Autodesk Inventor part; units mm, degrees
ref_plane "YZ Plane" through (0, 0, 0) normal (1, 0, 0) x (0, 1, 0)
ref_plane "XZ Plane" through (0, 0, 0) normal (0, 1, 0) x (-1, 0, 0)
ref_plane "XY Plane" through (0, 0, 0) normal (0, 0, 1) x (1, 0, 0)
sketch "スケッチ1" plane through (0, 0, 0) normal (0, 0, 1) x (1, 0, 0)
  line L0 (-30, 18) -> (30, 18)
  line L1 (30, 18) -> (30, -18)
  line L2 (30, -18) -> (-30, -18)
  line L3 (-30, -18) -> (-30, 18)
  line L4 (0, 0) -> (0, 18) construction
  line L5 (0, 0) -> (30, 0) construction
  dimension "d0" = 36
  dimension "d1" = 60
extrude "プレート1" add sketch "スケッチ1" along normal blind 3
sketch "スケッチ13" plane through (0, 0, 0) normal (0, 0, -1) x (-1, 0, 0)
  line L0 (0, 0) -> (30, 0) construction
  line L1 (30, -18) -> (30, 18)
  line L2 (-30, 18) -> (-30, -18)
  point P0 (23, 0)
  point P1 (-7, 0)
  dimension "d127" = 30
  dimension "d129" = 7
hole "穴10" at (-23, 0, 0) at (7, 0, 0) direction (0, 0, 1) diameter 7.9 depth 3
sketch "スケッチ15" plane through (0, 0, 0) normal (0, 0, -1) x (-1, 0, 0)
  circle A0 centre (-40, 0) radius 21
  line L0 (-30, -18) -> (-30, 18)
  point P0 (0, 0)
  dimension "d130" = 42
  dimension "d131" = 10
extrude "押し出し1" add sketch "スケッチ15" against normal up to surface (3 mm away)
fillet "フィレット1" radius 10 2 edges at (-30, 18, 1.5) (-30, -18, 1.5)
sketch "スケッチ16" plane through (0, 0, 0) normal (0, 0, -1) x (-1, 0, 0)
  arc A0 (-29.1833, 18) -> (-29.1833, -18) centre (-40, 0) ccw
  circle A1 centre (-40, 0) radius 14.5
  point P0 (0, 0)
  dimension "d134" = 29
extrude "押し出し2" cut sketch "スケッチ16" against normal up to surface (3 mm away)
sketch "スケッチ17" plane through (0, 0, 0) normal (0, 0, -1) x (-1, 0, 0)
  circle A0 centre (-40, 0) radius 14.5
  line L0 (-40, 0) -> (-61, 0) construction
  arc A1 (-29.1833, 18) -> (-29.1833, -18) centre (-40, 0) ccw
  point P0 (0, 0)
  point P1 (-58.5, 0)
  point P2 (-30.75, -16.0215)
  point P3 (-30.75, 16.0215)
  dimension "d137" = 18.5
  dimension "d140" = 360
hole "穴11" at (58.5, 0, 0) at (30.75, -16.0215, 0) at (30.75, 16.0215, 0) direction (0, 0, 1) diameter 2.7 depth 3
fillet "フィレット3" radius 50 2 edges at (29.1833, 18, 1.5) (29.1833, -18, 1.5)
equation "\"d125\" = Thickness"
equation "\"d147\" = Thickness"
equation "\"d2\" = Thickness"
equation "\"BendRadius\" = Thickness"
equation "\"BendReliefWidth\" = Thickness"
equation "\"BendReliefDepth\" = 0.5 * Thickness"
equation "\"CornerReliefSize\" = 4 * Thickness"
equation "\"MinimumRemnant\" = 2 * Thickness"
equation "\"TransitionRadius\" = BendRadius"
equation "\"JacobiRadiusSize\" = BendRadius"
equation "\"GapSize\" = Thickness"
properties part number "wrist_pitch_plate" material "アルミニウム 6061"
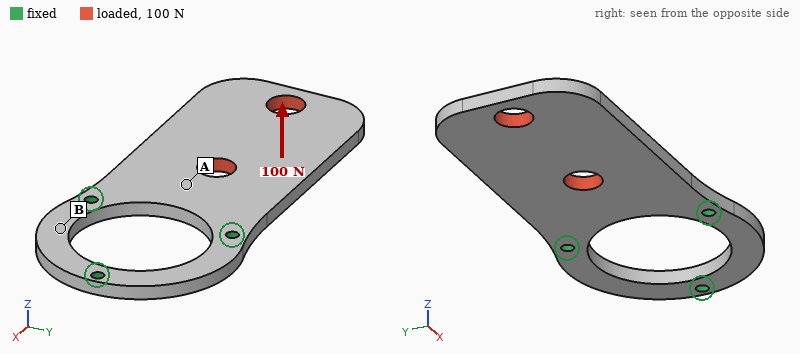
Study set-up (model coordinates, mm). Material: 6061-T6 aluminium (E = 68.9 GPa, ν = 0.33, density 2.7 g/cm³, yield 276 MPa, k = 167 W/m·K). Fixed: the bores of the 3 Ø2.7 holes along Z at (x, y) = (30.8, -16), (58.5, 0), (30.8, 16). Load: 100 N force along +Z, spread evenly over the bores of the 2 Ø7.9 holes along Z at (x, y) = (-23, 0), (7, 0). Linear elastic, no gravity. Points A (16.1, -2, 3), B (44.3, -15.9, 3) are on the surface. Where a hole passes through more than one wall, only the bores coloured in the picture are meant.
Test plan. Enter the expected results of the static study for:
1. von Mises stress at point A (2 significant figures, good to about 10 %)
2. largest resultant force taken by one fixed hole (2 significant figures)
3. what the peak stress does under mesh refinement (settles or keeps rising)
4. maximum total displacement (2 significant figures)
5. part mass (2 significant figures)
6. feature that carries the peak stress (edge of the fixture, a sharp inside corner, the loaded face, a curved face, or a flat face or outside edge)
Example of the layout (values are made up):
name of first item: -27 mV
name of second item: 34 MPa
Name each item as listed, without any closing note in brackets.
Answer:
von Mises stress at point A: 36 MPa
largest resultant force taken by one fixed hole: 51 N
what the peak stress does under mesh refinement: keeps rising
maximum total displacement: 1.0 mm
part mass: 20 g
feature that carries the peak stress: edge of the fixture
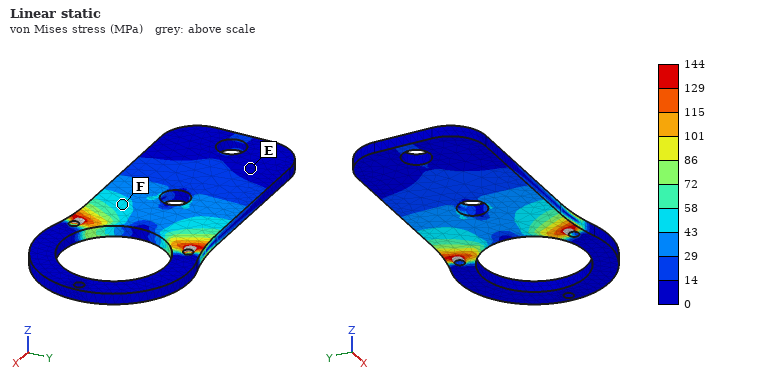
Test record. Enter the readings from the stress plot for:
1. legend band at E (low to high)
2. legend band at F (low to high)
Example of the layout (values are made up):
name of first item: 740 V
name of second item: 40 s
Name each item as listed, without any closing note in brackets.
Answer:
legend band at E: 0 to 14 MPa
legend band at F: 43 to 58 MPa
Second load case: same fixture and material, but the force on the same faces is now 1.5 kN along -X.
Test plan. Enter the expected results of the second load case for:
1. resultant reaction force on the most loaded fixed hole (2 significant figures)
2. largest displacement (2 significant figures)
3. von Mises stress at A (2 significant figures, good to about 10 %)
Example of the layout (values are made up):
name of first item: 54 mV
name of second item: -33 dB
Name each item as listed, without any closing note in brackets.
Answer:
resultant reaction force on the most loaded fixed hole: 800 N
largest displacement: 16 µm
von Mises stress at A: 8.4 MPa
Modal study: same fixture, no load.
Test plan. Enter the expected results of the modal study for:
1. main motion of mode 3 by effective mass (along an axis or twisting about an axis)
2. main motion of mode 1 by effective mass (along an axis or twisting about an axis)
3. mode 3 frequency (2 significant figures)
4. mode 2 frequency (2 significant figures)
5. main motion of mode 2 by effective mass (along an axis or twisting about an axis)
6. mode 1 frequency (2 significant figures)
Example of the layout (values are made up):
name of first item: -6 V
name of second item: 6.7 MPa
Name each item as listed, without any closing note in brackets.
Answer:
main motion of mode 3 by effective mass: along Z
main motion of mode 1 by effective mass: along Z
mode 3 frequency: 3900 Hz
mode 2 frequency: 2500 Hz
main motion of mode 2 by effective mass: twisting about X
mode 1 frequency: 590 Hz
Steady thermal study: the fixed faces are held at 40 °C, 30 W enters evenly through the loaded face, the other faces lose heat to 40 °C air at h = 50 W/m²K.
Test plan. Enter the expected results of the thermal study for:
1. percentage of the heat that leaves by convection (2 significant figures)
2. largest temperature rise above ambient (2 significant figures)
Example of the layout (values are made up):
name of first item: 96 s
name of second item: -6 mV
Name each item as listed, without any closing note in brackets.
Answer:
percentage of the heat that leaves by convection: 30 %
largest temperature rise above ambient: 66 K
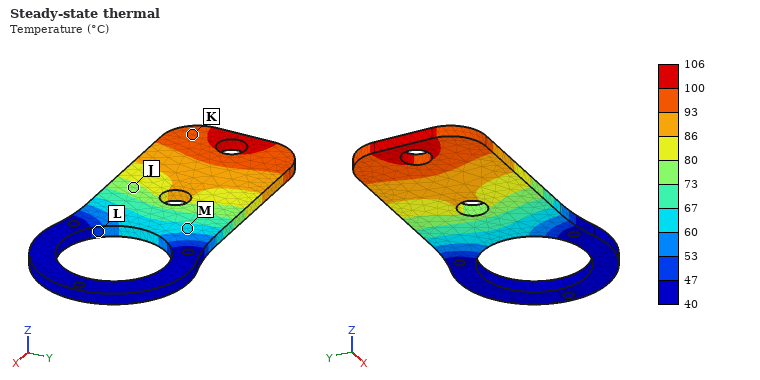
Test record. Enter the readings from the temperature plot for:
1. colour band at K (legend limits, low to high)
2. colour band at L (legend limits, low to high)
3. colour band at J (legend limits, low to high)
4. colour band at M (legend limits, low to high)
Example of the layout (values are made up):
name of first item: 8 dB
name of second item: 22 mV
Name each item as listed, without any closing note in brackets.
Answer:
colour band at K: 93 to 100 °C
colour band at L: 47 to 53 °C
colour band at J: 73 to 80 °C
colour band at M: 60 to 67 °C
